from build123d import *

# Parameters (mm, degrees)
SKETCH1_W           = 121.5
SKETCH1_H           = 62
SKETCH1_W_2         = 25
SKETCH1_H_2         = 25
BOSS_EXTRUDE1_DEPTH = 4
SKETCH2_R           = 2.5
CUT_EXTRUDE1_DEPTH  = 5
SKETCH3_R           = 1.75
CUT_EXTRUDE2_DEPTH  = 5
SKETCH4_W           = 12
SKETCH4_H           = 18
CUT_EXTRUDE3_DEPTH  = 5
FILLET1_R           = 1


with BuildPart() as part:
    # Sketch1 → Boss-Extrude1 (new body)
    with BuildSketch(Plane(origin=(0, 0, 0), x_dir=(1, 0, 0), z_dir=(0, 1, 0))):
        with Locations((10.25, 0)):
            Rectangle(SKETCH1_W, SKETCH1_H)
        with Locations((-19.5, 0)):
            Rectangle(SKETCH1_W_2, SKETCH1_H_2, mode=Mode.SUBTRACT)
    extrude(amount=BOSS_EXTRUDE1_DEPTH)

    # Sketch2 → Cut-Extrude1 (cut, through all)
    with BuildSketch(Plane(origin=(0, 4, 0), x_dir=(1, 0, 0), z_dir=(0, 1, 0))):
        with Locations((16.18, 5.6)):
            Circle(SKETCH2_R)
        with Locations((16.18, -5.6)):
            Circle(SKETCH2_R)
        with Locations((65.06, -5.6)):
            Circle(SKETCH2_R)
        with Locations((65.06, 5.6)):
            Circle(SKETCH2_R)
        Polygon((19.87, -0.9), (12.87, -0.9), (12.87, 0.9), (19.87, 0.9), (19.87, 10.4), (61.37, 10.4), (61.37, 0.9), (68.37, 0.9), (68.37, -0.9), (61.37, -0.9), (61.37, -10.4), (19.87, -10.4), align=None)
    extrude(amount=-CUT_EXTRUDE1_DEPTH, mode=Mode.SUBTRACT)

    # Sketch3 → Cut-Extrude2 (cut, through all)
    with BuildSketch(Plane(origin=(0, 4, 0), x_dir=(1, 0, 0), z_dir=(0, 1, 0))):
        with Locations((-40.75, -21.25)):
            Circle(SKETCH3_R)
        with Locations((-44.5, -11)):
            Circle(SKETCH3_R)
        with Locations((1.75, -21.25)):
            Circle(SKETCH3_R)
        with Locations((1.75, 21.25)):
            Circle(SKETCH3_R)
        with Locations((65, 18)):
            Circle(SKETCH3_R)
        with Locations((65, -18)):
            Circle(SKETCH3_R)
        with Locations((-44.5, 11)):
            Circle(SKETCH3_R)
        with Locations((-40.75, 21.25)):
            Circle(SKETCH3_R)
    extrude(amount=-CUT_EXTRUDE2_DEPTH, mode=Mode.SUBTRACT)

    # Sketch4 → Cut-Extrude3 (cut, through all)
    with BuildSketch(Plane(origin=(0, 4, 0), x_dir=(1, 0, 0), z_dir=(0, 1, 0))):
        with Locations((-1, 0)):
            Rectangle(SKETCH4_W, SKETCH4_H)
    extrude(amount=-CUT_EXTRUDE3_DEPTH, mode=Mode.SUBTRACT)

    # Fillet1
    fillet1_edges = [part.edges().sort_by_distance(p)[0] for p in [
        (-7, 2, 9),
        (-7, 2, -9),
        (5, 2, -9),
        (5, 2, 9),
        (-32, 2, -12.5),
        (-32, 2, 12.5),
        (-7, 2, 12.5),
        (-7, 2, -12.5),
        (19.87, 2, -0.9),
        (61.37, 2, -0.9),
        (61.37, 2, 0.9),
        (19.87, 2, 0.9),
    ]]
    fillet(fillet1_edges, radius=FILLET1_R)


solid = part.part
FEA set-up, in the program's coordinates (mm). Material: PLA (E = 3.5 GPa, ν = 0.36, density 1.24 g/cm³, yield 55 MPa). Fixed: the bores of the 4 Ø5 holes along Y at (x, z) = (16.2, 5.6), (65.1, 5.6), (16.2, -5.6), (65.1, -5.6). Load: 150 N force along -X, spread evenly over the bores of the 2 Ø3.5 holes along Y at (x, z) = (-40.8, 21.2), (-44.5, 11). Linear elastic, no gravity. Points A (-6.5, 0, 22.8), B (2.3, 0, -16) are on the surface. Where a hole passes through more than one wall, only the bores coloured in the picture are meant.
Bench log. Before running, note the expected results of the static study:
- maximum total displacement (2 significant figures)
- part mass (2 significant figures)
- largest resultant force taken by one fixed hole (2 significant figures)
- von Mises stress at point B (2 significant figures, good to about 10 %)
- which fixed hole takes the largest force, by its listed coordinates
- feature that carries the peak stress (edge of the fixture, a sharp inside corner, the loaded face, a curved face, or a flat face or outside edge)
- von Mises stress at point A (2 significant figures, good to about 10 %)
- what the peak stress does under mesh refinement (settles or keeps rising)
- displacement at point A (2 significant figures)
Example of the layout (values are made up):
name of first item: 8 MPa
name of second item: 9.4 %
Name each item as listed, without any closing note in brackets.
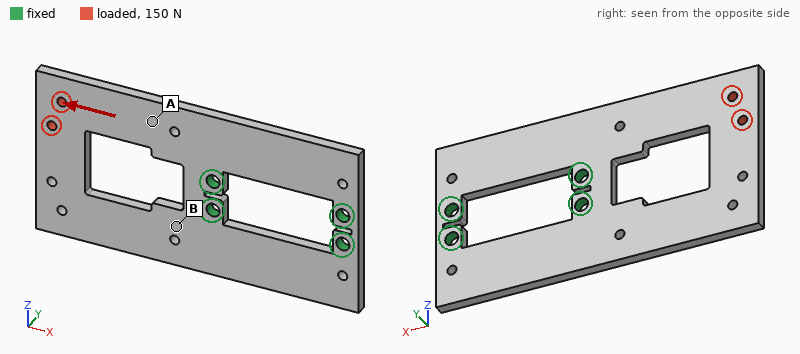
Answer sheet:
maximum total displacement: 63 µm
part mass: 28 g
largest resultant force taken by one fixed hole: 100 N
von Mises stress at point B: 0.44 MPa
which fixed hole takes the largest force, by its listed coordinates: (16.2, 5.6)
feature that carries the peak stress: edge of the fixture
von Mises stress at point A: 1.4 MPa
what the peak stress does under mesh refinement: keeps rising
displacement at point A: 38 µm
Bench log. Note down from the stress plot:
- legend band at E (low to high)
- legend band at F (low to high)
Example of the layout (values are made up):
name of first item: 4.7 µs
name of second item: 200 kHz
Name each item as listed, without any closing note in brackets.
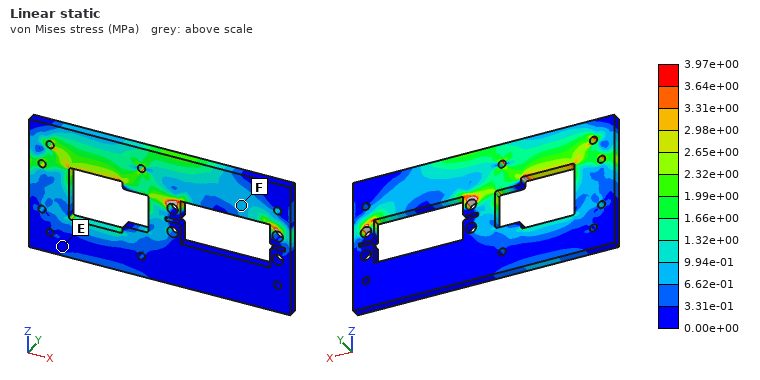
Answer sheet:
legend band at E: 0.00e+00 to 3.31e-01 MPa
legend band at F: 6.62e-01 to 9.94e-01 MPa
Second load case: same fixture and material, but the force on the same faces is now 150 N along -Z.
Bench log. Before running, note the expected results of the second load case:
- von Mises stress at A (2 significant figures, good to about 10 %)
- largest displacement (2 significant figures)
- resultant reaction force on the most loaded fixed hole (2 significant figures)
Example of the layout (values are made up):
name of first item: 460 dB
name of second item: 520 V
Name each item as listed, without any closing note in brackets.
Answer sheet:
von Mises stress at A: 2.9 MPa
largest displacement: 0.35 mm
resultant reaction force on the most loaded fixed hole: 140 N
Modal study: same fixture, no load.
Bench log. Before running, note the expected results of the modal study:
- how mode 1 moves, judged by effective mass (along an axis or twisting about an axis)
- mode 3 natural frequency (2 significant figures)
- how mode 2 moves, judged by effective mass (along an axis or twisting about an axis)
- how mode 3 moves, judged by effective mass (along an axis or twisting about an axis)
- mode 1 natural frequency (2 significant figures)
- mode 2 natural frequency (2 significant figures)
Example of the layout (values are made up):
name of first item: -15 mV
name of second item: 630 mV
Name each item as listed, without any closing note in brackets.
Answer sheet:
how mode 1 moves, judged by effective mass: along Y
mode 3 natural frequency: 1000 Hz
how mode 2 moves, judged by effective mass: twisting about X
how mode 3 moves, judged by effective mass: along Y
mode 1 natural frequency: 200 Hz
mode 2 natural frequency: 440 Hz
